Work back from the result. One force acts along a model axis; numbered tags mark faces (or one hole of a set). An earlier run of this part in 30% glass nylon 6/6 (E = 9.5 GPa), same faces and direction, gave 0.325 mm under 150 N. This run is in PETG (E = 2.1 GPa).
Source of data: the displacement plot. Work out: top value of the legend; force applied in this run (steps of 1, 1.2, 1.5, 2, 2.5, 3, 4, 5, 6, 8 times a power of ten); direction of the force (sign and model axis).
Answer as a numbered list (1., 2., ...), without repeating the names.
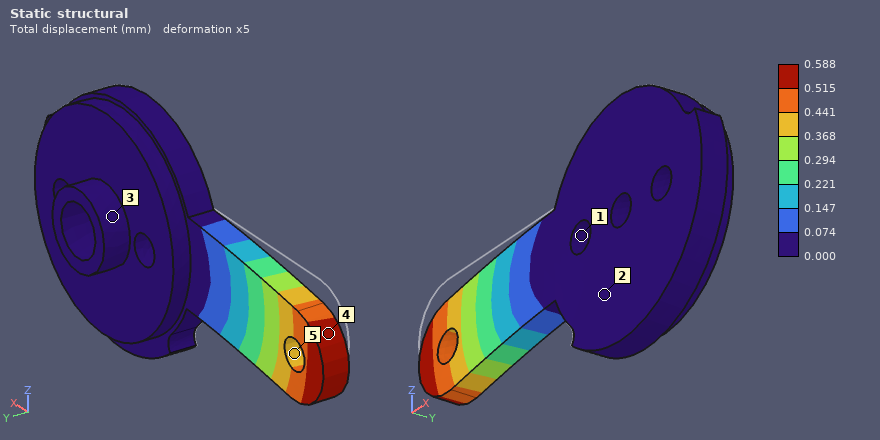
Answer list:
1. 0.588 mm
2. 60 N
3. -Z
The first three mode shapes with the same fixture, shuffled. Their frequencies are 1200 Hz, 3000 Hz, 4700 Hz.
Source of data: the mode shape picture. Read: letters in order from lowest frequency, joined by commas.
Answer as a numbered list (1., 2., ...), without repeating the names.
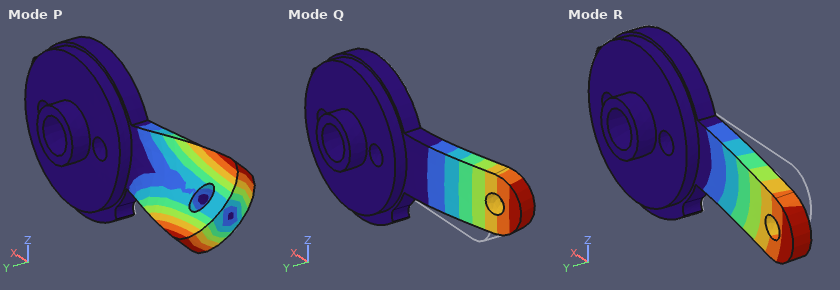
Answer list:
1. Q, R, P
